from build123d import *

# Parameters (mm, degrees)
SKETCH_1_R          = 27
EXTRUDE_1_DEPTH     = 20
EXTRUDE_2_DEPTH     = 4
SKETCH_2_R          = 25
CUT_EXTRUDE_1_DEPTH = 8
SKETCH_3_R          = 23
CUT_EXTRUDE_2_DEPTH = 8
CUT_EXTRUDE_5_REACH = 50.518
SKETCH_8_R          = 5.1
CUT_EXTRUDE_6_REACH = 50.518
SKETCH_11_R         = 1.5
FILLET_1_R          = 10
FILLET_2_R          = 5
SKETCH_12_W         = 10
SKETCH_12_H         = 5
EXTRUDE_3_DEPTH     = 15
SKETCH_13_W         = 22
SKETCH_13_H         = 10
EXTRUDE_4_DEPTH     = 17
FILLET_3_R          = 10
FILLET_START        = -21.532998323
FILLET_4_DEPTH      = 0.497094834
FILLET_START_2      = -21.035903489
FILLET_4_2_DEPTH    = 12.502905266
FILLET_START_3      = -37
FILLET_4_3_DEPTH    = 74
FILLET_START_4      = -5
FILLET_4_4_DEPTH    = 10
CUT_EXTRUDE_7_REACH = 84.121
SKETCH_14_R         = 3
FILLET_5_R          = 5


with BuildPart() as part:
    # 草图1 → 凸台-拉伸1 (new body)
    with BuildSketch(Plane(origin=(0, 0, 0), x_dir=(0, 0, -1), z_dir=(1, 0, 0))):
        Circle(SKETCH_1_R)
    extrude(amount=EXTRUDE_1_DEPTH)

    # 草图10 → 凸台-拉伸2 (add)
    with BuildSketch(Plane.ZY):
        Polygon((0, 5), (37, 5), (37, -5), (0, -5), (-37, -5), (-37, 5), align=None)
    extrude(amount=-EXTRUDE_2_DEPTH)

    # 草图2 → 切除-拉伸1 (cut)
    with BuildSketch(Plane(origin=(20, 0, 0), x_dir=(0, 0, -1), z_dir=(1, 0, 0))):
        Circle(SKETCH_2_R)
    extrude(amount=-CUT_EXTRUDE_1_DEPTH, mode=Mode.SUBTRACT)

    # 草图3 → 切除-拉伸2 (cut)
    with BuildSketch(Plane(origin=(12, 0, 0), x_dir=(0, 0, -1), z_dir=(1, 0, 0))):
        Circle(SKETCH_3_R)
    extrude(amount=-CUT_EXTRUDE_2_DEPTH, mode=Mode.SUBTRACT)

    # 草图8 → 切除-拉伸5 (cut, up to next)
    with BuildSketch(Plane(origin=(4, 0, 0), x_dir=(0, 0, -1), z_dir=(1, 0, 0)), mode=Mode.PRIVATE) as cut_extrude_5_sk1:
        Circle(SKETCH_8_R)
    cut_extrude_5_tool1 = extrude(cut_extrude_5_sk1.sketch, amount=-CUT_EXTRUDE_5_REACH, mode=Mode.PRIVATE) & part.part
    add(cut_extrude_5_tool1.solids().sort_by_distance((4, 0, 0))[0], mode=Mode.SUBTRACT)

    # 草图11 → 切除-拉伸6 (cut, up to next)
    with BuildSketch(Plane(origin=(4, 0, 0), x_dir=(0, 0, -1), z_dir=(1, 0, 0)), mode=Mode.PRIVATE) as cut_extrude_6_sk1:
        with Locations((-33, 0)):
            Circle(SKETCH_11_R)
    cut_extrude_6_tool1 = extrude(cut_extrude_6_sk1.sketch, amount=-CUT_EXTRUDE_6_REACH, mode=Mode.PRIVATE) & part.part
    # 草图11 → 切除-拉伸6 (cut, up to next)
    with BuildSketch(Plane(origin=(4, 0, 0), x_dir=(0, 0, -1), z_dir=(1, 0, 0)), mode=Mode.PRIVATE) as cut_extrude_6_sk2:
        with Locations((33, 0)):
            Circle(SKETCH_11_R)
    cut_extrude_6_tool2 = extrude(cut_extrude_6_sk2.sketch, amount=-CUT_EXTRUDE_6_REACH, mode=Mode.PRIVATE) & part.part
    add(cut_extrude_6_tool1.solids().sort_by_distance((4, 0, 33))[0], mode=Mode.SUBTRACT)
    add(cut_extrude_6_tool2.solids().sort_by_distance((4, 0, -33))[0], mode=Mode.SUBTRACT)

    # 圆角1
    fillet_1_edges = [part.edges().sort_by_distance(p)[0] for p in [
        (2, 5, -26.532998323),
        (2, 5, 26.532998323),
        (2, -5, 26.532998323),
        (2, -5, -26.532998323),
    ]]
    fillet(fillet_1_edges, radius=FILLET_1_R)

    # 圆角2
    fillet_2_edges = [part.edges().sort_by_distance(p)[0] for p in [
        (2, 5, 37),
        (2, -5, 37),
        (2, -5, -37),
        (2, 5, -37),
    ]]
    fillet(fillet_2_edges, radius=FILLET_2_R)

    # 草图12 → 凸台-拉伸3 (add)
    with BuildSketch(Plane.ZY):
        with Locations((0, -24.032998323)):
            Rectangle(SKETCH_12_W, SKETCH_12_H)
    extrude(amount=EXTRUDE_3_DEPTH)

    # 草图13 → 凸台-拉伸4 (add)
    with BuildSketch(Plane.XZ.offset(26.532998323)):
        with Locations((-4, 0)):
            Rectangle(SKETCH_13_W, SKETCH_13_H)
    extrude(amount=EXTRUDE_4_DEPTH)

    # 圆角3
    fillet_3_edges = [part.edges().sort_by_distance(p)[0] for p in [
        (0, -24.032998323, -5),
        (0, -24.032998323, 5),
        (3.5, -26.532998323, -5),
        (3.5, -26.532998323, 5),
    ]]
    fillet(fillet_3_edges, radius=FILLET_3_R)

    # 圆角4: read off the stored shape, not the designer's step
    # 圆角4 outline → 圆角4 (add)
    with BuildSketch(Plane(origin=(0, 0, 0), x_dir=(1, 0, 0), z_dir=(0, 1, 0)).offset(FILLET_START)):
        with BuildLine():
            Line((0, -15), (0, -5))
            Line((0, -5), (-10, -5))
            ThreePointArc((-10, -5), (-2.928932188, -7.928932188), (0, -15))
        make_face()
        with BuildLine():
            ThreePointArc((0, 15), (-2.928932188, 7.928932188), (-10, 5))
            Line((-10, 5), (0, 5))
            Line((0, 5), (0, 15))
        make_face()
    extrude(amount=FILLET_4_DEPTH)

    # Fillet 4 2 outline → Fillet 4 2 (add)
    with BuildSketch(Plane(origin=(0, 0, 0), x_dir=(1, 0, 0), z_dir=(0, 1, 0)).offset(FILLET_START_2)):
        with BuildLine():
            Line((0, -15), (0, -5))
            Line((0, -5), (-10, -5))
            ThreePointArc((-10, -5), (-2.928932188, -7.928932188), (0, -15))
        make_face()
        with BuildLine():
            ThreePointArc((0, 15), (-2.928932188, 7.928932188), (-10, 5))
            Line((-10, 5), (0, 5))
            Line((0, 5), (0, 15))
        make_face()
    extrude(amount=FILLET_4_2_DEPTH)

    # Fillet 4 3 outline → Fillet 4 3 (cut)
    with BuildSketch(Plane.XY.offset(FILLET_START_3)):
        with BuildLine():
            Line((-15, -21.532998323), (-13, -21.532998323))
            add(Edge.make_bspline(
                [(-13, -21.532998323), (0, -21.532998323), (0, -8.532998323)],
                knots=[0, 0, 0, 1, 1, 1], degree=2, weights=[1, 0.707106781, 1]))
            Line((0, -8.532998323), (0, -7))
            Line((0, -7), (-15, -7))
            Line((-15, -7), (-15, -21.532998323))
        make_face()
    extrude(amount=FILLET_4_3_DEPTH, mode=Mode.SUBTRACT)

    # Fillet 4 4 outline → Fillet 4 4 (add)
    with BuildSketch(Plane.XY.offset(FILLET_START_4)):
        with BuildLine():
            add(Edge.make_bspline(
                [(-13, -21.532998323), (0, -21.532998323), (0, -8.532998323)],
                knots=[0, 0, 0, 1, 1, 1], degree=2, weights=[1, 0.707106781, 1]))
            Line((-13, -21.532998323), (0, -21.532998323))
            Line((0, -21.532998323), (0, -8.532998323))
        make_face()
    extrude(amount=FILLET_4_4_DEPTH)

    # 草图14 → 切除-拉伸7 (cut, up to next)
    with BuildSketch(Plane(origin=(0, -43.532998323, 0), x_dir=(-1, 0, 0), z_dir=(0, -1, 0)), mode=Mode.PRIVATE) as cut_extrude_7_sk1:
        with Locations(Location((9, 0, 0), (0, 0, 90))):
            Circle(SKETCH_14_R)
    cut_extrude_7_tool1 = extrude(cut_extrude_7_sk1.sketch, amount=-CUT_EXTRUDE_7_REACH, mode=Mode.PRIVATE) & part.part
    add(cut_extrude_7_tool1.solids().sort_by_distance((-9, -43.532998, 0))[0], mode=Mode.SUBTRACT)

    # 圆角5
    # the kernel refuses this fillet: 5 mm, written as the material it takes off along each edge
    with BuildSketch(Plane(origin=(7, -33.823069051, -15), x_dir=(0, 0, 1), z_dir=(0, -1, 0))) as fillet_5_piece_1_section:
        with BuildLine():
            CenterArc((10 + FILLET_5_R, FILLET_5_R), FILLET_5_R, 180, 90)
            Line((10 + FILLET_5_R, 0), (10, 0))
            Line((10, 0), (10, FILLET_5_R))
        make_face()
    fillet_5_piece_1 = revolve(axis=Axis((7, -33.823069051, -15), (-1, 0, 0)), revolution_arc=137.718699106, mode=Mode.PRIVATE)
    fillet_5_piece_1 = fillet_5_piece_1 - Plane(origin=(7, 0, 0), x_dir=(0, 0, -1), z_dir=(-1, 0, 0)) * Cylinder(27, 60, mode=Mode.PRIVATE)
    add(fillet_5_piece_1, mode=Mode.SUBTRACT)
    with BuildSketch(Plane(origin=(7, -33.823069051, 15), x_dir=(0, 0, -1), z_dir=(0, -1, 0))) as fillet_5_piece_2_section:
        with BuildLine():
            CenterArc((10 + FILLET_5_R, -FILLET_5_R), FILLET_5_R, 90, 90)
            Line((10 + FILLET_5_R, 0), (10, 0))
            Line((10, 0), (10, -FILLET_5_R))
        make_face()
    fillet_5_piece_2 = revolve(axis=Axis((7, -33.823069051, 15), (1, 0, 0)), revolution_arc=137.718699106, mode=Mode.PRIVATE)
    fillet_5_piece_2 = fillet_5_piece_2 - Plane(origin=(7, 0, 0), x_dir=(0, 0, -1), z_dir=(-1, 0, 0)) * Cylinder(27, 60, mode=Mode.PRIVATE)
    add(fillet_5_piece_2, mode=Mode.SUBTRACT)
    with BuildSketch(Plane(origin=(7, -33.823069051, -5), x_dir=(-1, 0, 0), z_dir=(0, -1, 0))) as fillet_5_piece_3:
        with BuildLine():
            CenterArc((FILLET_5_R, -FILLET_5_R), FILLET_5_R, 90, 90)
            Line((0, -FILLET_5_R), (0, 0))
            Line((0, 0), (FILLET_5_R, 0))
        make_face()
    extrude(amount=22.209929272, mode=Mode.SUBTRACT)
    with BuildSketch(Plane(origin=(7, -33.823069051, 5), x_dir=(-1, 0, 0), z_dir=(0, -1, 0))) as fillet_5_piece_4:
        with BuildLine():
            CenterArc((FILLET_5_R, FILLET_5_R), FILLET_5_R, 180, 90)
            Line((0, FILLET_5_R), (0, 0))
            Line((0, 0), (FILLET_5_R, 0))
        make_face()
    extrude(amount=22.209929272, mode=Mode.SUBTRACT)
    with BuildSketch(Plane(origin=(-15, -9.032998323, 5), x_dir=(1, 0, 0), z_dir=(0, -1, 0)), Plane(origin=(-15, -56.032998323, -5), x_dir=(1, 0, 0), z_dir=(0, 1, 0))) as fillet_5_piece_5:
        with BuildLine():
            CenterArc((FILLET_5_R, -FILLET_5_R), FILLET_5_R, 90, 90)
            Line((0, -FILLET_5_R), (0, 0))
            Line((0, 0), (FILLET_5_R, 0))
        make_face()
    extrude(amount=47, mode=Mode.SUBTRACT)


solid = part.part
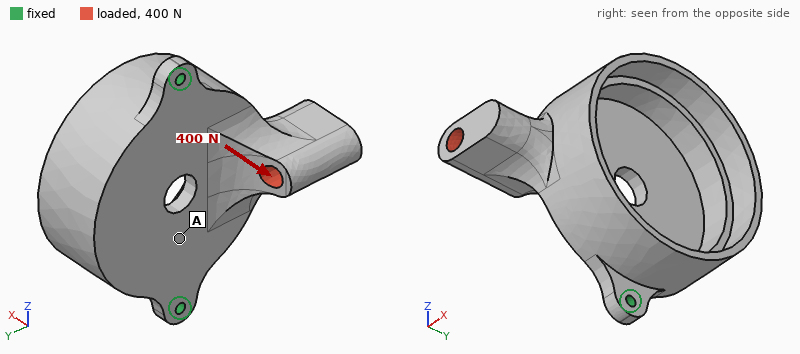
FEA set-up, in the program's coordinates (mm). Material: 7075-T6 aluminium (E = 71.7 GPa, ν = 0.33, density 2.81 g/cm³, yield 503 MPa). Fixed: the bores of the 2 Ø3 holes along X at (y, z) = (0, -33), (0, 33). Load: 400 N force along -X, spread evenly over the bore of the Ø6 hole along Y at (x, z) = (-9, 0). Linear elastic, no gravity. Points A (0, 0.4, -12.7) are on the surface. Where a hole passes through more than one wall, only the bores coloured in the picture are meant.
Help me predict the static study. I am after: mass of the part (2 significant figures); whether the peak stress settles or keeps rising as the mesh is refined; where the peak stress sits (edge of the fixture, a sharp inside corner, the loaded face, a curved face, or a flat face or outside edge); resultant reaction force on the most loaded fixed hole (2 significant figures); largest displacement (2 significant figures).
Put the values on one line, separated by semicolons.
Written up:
61 g; keeps rising; edge of the fixture; 200 N; 0.44 mm
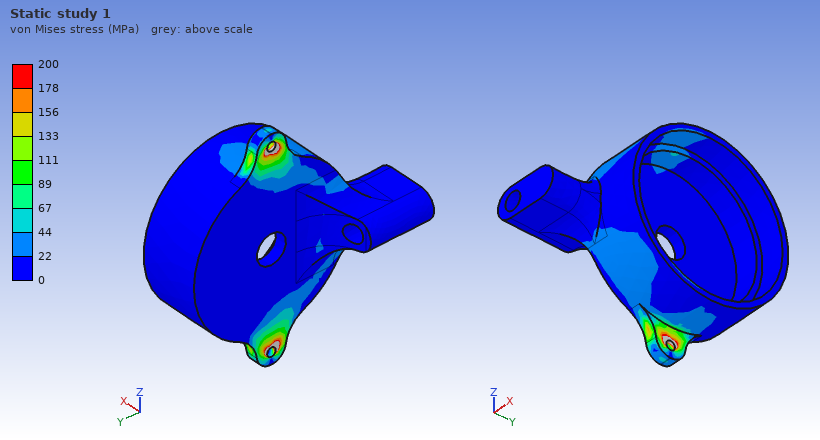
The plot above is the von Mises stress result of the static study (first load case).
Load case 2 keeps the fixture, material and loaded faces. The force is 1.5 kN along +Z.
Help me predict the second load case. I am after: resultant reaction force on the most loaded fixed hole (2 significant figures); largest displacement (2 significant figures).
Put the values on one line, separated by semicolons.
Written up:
1.1 kN; 88 µm
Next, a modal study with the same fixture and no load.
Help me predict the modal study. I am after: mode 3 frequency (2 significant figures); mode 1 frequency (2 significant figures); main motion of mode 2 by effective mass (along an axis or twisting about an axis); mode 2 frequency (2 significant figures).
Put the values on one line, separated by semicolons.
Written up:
6700 Hz; 1200 Hz; along X; 3200 Hz
